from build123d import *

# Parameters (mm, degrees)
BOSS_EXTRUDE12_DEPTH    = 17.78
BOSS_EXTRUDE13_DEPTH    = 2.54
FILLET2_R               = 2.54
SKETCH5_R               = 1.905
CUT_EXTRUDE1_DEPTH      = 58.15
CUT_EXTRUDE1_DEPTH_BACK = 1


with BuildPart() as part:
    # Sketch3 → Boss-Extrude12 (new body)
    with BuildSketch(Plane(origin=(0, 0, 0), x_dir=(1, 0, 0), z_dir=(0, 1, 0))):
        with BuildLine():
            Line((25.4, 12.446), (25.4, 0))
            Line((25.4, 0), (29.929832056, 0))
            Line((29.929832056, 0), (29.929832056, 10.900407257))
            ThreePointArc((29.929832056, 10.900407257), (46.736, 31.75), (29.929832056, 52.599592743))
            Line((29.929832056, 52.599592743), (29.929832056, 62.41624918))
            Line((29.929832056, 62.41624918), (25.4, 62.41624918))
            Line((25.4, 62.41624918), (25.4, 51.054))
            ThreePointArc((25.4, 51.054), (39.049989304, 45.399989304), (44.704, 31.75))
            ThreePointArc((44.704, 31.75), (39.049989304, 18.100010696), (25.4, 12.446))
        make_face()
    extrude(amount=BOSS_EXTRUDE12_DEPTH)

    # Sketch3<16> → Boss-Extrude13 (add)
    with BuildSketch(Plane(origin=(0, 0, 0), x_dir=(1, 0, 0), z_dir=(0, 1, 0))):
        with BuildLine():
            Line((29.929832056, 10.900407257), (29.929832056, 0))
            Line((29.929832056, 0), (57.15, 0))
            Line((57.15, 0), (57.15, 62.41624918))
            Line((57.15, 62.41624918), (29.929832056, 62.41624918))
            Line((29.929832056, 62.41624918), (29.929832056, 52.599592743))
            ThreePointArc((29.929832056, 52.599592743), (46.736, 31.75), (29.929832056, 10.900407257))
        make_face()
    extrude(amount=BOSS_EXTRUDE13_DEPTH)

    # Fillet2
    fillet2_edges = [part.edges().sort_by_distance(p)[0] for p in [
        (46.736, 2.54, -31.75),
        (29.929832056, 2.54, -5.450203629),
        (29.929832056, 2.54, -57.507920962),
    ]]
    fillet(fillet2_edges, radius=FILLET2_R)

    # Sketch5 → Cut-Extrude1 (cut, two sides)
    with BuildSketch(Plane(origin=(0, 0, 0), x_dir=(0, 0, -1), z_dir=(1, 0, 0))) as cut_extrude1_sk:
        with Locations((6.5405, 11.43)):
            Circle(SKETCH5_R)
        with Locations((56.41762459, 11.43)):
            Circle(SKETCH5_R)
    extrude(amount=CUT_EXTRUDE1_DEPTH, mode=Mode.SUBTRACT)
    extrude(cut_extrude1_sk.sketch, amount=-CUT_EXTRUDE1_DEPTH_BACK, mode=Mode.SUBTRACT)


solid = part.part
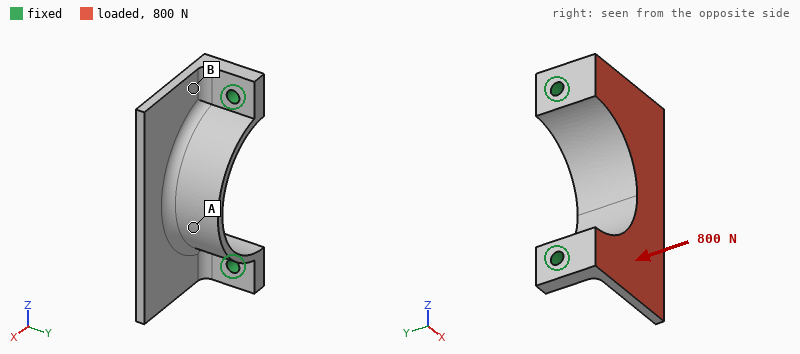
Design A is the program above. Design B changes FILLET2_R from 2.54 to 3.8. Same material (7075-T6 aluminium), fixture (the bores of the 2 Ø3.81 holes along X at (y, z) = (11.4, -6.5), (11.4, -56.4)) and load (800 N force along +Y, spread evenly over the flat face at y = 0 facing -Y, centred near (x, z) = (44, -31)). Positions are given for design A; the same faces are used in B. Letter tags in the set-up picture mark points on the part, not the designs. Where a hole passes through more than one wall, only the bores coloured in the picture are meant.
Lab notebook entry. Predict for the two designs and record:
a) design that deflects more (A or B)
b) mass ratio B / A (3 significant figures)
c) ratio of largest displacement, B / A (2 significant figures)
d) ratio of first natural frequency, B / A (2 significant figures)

A
1.02
0.91
1.0
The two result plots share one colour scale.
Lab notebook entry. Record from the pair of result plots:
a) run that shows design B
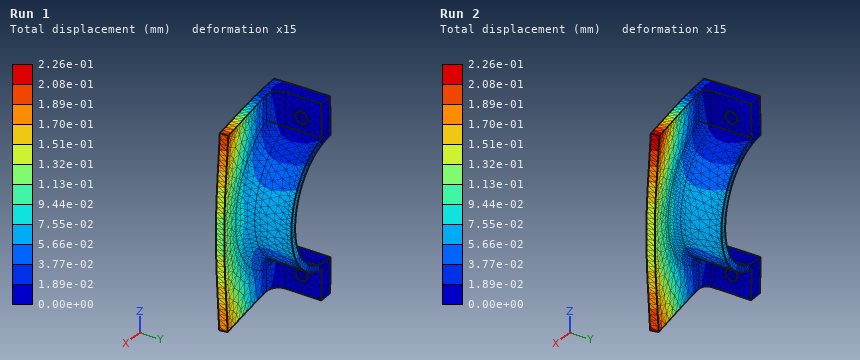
Run 1
